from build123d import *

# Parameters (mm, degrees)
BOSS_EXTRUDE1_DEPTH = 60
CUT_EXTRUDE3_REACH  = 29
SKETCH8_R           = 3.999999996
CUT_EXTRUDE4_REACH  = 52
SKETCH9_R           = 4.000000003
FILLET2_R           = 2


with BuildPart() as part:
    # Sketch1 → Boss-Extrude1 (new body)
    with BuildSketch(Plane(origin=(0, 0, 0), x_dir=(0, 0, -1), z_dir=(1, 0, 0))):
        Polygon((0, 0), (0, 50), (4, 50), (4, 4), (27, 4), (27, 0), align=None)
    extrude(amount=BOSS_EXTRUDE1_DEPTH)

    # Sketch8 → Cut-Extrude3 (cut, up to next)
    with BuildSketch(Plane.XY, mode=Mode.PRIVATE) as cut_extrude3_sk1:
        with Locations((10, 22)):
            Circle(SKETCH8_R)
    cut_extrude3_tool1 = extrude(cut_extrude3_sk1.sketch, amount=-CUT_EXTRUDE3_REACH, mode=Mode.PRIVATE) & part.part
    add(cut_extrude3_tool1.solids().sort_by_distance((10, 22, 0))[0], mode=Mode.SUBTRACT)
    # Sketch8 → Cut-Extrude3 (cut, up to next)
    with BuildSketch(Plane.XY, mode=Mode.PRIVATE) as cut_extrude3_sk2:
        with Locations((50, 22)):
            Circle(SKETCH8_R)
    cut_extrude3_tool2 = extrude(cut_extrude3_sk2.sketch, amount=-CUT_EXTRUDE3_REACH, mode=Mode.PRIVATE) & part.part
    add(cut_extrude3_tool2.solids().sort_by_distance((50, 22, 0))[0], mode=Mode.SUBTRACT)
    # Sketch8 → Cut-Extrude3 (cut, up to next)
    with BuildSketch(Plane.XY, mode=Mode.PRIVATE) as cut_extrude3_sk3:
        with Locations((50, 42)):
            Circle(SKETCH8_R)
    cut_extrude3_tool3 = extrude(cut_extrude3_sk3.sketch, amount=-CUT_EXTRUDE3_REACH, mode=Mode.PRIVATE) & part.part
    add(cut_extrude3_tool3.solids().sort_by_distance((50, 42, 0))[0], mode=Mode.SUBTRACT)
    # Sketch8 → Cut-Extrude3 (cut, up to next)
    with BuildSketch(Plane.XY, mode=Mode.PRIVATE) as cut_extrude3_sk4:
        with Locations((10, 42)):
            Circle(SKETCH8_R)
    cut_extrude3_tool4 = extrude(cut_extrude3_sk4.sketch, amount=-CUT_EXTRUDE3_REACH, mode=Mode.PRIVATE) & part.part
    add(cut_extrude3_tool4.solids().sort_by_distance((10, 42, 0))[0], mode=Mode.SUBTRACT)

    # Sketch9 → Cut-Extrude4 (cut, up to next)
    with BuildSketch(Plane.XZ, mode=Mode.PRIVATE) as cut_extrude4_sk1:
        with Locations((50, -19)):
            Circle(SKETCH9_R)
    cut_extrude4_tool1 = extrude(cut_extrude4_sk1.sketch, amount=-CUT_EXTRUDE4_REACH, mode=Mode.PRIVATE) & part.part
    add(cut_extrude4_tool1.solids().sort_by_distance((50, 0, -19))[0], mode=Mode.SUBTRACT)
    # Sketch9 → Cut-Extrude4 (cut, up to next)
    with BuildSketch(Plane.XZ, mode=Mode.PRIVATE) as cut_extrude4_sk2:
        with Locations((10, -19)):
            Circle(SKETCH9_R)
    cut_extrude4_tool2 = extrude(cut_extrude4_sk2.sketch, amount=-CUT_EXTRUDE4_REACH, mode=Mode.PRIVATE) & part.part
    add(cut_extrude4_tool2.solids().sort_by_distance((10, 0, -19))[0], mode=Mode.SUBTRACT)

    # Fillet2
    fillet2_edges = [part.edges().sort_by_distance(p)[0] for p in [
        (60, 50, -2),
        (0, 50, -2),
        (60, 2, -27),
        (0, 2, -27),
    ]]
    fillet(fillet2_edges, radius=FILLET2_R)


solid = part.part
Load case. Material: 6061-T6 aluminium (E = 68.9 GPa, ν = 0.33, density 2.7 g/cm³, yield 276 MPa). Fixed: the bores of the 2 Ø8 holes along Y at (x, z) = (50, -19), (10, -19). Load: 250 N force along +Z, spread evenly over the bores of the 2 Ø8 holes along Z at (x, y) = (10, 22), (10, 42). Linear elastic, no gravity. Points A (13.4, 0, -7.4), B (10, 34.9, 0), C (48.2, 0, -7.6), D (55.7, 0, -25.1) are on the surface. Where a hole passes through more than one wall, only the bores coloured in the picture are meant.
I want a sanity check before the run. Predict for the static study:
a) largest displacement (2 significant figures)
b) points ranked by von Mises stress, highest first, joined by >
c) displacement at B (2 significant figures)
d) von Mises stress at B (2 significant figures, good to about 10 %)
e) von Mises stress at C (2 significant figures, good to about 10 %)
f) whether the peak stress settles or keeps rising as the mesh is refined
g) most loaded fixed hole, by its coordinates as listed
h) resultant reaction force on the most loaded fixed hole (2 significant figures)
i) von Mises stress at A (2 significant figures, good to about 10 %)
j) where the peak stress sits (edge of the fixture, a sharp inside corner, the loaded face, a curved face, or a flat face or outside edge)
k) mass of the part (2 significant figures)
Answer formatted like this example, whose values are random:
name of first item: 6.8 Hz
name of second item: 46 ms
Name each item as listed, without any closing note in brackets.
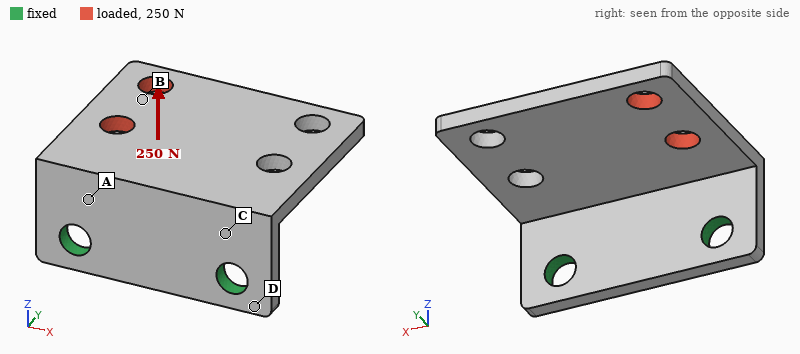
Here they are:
largest displacement: 0.54 mm
points ranked by von Mises stress, highest first, joined by >: A > C > B > D
displacement at B: 0.33 mm
von Mises stress at B: 18 MPa
von Mises stress at C: 33 MPa
whether the peak stress settles or keeps rising as the mesh is refined: keeps rising
most loaded fixed hole, by its coordinates as listed: (10, -19)
resultant reaction force on the most loaded fixed hole: 240 N
von Mises stress at A: 53 MPa
where the peak stress sits: edge of the fixture
mass of the part: 44 g
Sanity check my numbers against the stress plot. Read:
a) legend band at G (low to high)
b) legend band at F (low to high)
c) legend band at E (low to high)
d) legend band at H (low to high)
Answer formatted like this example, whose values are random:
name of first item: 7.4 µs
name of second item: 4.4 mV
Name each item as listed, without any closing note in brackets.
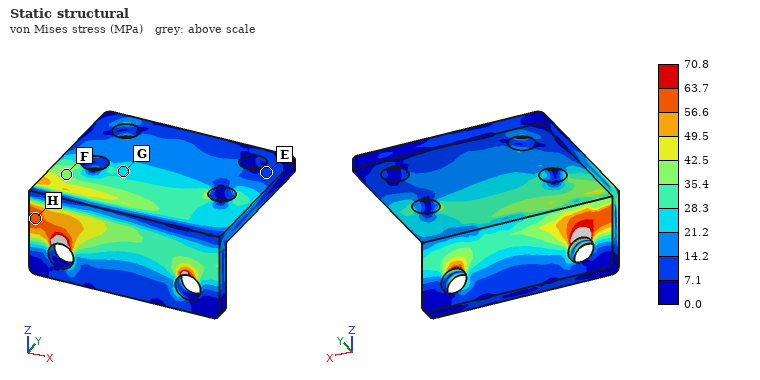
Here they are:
legend band at G: 21.2 to 28.3 MPa
legend band at F: 35.4 to 42.5 MPa
legend band at E: 7.1 to 14.2 MPa
legend band at H: 56.6 to 63.7 MPa
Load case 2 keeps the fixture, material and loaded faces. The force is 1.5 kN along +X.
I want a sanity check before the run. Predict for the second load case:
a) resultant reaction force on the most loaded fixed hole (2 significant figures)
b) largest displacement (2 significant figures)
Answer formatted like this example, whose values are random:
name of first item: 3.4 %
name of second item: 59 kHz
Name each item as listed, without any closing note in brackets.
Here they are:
resultant reaction force on the most loaded fixed hole: 1.4 kN
largest displacement: 0.27 mm
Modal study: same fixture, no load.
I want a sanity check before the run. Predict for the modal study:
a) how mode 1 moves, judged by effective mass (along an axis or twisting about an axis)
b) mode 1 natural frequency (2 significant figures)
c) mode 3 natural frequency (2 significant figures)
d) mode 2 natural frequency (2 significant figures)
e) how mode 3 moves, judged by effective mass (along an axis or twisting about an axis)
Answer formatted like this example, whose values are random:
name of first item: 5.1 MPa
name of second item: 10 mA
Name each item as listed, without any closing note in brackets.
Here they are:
how mode 1 moves, judged by effective mass: along Z
mode 1 natural frequency: 1000 Hz
mode 3 natural frequency: 3600 Hz
mode 2 natural frequency: 2400 Hz
how mode 3 moves, judged by effective mass: along X
